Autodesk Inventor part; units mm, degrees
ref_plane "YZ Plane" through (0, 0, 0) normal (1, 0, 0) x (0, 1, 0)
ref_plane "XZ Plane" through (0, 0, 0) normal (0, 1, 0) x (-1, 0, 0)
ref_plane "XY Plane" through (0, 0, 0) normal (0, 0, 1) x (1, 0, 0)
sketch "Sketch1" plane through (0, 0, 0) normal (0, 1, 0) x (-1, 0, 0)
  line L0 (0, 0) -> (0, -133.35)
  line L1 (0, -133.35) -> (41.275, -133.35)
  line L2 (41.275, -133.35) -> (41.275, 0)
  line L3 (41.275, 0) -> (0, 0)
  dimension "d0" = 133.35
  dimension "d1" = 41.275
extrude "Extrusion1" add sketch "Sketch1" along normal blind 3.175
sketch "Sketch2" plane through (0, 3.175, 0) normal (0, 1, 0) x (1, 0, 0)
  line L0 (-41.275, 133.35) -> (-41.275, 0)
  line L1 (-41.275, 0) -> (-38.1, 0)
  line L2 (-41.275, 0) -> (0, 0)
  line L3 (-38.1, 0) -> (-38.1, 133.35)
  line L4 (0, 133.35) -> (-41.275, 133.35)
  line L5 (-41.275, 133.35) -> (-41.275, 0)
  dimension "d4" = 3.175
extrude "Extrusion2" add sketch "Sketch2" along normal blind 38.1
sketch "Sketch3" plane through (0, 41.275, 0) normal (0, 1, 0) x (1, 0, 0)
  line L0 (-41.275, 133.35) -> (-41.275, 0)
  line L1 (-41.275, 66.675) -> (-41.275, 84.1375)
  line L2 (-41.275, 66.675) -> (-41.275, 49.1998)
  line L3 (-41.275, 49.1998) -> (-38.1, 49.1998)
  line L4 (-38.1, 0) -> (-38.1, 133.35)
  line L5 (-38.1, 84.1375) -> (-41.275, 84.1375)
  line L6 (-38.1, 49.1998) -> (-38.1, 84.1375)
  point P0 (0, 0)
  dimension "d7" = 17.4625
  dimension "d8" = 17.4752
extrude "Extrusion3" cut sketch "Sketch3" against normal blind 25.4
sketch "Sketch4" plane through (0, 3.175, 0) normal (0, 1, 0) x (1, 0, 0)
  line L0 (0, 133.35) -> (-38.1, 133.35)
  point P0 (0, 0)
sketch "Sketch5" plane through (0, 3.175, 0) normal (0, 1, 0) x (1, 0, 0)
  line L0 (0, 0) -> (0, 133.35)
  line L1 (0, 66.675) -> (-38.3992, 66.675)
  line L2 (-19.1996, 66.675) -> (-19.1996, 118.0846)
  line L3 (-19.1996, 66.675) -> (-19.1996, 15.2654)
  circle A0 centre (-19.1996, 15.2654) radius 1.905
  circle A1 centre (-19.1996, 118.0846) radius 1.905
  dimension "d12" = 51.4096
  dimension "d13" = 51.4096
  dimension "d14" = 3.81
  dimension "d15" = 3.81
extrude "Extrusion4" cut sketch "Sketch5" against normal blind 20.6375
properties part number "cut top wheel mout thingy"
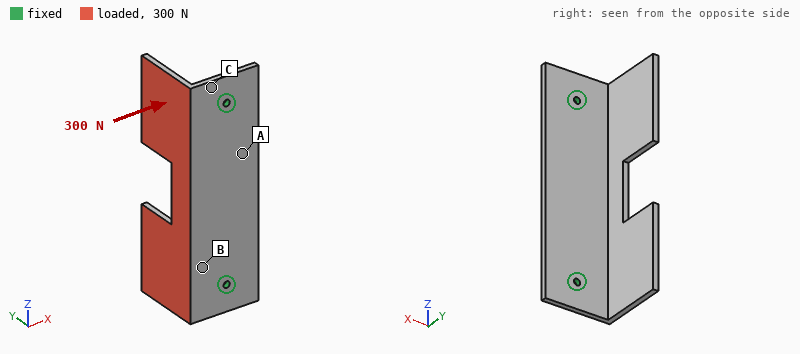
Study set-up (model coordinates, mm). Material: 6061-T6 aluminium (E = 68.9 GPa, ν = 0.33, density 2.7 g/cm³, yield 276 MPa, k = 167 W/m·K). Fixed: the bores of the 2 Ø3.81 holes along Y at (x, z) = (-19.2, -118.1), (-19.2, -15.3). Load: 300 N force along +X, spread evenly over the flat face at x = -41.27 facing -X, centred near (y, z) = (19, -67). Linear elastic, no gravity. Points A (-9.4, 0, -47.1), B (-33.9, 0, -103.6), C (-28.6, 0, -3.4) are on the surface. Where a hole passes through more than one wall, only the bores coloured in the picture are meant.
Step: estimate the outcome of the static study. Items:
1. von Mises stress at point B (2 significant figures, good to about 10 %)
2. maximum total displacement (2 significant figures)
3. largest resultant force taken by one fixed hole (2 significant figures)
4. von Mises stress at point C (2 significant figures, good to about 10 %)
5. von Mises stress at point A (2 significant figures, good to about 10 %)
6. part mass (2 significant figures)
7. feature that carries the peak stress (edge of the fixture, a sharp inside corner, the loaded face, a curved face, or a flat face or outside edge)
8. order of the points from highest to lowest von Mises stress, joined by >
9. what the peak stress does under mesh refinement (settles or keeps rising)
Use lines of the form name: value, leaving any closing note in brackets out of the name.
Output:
von Mises stress at point B: 23 MPa
maximum total displacement: 0.36 mm
largest resultant force taken by one fixed hole: 150 N
von Mises stress at point C: 32 MPa
von Mises stress at point A: 8.9 MPa
part mass: 83 g
feature that carries the peak stress: edge of the fixture
order of the points from highest to lowest von Mises stress, joined by >: C > B > A
what the peak stress does under mesh refinement: keeps rising
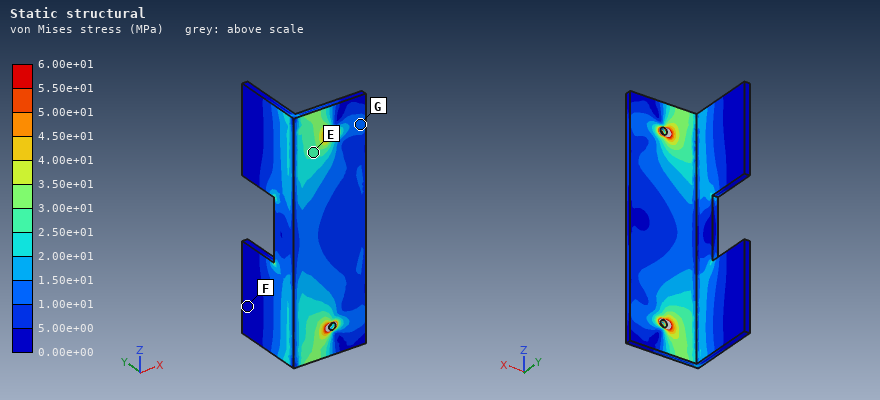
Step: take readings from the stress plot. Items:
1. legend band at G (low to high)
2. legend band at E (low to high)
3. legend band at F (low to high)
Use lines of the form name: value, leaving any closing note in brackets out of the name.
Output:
legend band at G: 1.00e+01 to 1.50e+01 MPa
legend band at E: 2.50e+01 to 3.00e+01 MPa
legend band at F: 0.00e+00 to 5.00e+00 MPa
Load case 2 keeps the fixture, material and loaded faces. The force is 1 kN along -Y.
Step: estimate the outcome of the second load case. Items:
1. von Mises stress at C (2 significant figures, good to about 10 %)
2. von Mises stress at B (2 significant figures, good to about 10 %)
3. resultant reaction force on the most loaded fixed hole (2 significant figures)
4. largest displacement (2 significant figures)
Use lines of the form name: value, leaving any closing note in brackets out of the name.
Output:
von Mises stress at C: 87 MPa
von Mises stress at B: 38 MPa
resultant reaction force on the most loaded fixed hole: 530 N
largest displacement: 0.80 mm
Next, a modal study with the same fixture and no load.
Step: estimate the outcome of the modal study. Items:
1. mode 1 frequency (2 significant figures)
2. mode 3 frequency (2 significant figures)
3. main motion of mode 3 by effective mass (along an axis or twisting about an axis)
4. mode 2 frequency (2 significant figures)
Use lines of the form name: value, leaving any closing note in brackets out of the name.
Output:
mode 1 frequency: 820 Hz
mode 3 frequency: 1800 Hz
main motion of mode 3 by effective mass: along Y
mode 2 frequency: 1100 Hz
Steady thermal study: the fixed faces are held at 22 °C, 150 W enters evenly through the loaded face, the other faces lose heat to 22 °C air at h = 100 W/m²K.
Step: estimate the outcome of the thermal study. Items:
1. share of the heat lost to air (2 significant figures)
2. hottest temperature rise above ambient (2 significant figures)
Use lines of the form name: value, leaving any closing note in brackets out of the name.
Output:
share of the heat lost to air: 48 %
hottest temperature rise above ambient: 84 K
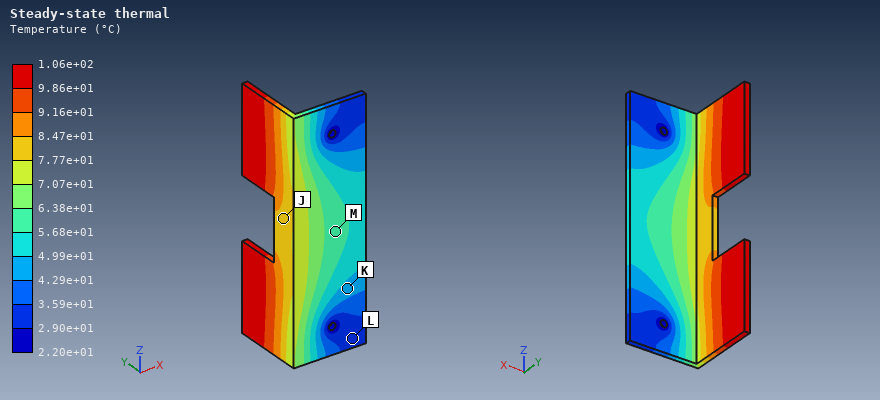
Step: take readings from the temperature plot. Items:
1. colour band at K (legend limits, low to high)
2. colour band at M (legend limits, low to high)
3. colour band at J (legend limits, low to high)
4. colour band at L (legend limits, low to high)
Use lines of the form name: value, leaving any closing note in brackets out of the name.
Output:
colour band at K: 4.29e+01 to 4.99e+01 °C
colour band at M: 5.68e+01 to 6.38e+01 °C
colour band at J: 7.77e+01 to 8.47e+01 °C
colour band at L: 2.90e+01 to 3.59e+01 °C
